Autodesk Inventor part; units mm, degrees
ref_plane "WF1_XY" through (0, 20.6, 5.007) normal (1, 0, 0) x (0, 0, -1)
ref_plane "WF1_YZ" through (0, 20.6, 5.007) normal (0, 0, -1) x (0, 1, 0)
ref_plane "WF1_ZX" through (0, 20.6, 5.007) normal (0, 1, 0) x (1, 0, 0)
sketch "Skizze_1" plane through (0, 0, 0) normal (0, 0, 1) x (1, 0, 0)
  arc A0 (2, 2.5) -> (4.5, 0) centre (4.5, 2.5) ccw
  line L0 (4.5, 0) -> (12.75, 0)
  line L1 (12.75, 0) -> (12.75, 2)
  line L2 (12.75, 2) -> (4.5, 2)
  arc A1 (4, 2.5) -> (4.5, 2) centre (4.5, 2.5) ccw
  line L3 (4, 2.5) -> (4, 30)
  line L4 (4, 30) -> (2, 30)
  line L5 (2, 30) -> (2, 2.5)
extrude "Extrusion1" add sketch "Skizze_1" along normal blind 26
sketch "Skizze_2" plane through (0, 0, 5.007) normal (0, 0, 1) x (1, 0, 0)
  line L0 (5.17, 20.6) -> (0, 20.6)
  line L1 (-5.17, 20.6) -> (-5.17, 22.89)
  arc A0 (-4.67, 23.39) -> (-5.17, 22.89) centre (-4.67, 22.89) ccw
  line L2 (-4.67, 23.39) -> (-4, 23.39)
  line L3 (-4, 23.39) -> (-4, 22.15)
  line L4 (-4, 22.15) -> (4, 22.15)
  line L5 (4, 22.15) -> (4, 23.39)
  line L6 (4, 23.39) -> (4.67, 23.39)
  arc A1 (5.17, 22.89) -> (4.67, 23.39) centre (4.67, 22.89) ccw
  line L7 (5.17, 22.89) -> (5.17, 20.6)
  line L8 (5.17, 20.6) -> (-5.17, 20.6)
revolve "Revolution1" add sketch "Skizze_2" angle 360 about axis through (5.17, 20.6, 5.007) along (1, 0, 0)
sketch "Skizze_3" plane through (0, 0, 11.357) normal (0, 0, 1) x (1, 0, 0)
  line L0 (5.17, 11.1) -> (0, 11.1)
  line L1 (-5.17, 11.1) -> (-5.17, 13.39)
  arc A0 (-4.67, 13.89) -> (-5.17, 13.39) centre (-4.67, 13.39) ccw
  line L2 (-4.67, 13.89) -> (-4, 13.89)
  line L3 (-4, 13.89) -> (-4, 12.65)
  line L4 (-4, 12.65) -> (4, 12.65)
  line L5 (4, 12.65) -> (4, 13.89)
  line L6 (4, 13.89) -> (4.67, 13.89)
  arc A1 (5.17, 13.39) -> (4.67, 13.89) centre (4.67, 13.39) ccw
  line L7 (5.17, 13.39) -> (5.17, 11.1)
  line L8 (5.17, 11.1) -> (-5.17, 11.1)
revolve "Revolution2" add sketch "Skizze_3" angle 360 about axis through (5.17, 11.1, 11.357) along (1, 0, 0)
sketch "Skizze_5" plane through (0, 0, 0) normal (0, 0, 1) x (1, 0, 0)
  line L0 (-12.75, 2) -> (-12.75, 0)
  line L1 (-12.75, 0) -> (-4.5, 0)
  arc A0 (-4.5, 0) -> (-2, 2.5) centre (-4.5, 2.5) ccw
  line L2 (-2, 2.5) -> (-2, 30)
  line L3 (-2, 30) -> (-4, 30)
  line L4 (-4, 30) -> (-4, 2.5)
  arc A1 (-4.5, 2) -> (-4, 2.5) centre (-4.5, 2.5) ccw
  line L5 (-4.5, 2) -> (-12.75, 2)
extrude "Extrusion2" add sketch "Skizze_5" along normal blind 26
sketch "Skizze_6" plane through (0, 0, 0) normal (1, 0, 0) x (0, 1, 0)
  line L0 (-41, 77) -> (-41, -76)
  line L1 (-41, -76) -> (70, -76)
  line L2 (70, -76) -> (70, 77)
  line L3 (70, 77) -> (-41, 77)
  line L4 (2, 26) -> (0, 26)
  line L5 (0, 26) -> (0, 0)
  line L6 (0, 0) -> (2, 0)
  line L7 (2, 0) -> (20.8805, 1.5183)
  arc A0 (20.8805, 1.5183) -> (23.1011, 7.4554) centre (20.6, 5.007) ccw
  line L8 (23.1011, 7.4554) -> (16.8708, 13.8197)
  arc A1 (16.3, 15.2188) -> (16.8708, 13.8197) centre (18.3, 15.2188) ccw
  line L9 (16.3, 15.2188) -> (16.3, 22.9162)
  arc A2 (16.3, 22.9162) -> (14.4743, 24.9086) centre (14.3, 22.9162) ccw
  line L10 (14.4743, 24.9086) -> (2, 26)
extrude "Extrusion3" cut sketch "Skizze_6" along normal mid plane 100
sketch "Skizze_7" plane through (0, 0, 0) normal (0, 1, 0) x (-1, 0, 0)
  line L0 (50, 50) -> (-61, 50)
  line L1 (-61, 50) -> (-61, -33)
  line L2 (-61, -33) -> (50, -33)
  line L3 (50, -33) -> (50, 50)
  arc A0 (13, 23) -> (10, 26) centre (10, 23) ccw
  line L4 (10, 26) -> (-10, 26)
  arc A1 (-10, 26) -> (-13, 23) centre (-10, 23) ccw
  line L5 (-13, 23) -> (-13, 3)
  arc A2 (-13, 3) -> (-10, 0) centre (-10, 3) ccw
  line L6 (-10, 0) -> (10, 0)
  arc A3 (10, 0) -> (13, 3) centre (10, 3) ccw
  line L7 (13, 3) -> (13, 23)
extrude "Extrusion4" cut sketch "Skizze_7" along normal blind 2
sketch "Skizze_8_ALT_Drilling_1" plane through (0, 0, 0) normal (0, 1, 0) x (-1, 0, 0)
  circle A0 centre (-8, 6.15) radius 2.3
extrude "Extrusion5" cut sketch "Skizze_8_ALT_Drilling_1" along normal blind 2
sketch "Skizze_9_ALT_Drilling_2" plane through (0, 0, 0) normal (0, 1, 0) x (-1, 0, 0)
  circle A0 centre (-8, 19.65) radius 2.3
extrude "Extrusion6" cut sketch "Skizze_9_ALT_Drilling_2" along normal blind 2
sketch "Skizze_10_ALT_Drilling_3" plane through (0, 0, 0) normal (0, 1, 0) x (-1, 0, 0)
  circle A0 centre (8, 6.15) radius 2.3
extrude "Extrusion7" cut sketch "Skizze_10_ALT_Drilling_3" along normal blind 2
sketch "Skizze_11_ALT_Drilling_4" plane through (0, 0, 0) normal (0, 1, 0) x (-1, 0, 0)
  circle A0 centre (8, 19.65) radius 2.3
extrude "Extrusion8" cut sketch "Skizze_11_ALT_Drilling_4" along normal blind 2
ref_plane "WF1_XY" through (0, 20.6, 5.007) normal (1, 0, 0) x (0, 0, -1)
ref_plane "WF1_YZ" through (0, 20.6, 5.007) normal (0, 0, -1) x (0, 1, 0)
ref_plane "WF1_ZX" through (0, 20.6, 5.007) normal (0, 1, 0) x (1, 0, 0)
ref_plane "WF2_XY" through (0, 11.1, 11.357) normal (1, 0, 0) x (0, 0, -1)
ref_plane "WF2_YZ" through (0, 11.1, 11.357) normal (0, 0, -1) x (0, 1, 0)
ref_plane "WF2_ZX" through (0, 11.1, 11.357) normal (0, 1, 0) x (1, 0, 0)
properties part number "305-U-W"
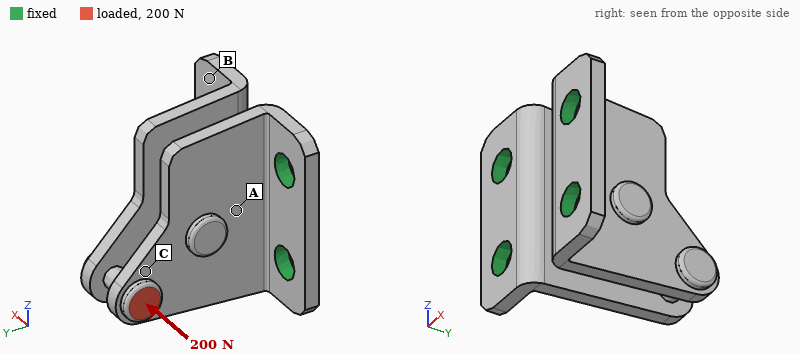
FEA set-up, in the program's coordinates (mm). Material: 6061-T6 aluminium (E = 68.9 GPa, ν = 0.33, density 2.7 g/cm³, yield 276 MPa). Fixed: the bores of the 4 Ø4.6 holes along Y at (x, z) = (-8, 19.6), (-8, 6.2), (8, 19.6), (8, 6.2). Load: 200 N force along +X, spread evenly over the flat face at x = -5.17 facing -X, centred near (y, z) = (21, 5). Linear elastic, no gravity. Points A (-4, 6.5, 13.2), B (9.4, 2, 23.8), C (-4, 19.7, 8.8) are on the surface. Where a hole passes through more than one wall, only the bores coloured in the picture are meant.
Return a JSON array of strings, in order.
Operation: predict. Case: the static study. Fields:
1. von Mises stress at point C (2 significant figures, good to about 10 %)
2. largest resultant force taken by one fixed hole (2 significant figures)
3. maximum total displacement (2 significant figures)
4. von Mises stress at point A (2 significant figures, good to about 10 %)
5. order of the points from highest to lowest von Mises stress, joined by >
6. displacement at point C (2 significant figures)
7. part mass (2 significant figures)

["22 MPa", "200 N", "85 µm", "36 MPa", "A > C > B", "63 µm", "7.5 g"]
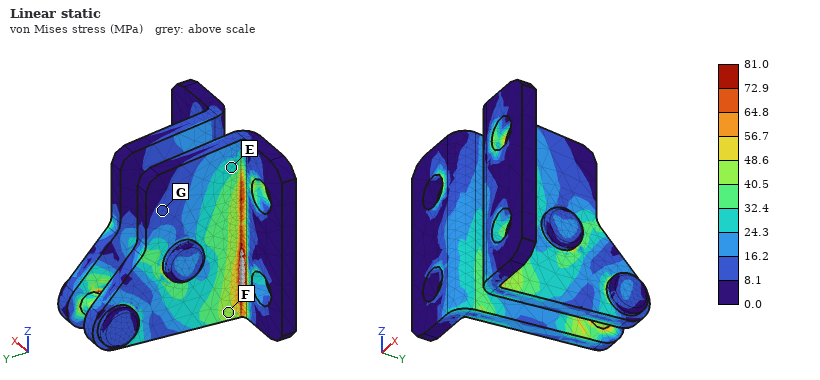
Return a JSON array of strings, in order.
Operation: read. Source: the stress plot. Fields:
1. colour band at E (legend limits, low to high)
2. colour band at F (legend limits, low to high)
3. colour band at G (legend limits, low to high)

["24.3 to 32.4 MPa", "40.5 to 48.6 MPa", "8.1 to 16.2 MPa"]
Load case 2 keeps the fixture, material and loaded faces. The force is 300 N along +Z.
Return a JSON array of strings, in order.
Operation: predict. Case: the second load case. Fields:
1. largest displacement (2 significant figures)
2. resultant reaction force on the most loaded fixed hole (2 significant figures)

["66 µm", "360 N"]
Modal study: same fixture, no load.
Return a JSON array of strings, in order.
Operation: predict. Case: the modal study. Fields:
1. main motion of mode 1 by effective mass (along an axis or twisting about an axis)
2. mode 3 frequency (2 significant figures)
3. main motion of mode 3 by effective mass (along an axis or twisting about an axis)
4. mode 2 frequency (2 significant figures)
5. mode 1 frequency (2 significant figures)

["along X", "12 kHz", "along Z", "9900 Hz", "7200 Hz"]
